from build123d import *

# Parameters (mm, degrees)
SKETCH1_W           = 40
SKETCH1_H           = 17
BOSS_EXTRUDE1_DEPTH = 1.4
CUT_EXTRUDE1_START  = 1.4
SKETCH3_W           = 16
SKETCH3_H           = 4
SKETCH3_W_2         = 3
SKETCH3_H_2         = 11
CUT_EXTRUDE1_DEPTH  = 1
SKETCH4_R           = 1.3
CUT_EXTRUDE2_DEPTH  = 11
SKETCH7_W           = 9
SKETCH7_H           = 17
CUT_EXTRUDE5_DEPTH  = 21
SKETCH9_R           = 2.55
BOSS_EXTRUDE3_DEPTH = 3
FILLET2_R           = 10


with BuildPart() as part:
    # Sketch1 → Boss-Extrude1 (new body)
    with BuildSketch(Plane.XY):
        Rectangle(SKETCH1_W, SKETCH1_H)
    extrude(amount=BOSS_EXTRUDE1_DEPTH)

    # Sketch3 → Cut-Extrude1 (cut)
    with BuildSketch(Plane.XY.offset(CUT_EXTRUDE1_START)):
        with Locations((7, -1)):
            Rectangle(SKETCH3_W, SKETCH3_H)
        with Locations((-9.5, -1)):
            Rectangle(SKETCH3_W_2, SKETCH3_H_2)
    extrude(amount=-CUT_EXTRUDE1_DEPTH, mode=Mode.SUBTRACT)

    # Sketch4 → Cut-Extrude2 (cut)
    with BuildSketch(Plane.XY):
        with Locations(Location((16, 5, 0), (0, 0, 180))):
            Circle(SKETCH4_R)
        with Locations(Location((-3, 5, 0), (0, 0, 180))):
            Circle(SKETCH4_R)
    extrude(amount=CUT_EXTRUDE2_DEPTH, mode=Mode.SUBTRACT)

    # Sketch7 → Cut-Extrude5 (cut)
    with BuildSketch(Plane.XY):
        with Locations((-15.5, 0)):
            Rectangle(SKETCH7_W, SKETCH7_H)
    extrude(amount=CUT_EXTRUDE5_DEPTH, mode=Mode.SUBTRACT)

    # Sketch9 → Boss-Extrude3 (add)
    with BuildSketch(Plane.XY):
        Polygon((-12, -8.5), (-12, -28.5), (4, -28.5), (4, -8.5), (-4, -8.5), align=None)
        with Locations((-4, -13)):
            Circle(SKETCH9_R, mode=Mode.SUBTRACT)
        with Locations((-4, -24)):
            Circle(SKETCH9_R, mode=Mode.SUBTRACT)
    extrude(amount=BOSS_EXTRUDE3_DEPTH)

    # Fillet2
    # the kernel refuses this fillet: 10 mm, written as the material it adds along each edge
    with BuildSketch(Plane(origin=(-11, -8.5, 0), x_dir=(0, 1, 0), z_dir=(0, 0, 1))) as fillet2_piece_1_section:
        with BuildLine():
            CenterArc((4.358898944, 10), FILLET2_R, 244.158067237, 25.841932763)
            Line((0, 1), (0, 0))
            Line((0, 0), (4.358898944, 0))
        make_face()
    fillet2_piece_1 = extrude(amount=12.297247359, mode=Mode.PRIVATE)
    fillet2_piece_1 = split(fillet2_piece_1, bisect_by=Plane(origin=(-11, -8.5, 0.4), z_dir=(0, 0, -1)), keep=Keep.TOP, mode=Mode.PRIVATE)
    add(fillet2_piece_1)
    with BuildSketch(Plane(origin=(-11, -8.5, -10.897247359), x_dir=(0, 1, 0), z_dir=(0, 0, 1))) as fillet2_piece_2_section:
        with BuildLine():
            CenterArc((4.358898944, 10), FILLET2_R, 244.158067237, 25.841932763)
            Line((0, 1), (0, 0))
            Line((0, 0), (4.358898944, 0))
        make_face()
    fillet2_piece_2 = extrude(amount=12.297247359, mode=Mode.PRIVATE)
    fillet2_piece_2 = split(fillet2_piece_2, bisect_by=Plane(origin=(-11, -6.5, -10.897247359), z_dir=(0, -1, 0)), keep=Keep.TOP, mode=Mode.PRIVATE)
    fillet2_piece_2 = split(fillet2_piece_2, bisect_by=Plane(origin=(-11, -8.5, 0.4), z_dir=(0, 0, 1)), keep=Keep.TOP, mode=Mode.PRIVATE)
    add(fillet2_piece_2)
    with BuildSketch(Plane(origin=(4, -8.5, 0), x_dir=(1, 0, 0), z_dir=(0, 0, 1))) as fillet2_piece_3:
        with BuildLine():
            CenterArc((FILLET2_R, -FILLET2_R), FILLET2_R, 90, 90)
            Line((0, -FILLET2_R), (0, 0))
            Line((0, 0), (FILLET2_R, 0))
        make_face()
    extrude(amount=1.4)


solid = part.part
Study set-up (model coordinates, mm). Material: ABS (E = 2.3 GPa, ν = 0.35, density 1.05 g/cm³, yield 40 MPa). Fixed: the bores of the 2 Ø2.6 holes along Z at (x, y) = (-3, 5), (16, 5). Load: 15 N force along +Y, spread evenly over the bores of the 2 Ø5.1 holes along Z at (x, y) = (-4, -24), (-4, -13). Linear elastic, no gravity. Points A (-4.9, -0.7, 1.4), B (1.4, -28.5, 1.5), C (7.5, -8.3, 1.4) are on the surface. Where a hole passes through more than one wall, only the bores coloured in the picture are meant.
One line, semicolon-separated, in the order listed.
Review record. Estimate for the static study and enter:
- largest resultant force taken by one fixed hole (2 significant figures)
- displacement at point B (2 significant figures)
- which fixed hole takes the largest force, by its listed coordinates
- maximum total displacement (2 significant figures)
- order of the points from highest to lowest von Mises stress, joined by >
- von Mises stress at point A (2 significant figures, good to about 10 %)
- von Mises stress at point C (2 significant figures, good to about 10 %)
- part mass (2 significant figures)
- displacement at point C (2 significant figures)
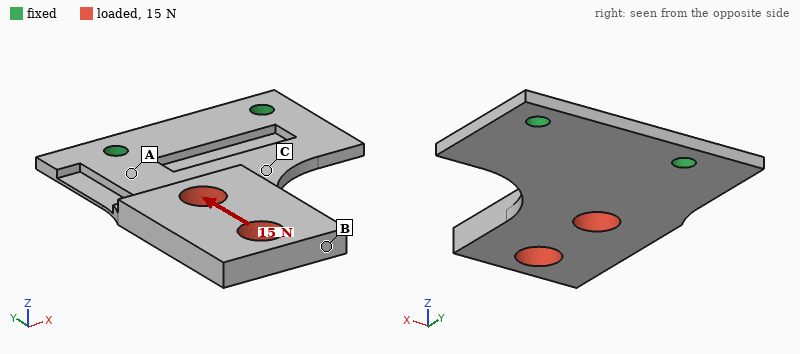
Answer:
15 N; 0.56 mm; (-3, 5); 0.59 mm; A > C > B; 4.3 MPa; 1.6 MPa; 1.6 g; 0.12 mm
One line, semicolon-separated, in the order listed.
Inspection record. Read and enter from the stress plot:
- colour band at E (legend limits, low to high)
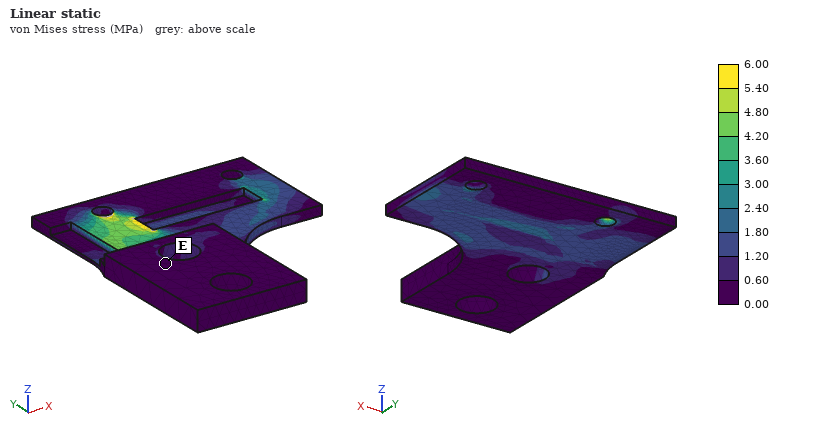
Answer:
0.00 to 0.60 MPa
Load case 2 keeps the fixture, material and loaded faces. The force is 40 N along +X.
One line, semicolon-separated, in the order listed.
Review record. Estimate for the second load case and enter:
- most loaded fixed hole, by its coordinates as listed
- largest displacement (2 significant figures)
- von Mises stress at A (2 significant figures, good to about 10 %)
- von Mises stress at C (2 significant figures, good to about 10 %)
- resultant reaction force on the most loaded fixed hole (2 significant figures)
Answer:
(16, 5); 0.54 mm; 3.5 MPa; 8.7 MPa; 52 N
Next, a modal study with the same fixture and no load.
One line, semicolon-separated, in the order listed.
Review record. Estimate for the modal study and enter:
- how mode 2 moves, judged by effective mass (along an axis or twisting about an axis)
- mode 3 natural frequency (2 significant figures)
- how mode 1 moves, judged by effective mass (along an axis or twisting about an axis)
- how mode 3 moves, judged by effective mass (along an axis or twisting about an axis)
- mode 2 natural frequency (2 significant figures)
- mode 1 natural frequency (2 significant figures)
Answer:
twisting about Y; 2000 Hz; along Z; along Z; 1200 Hz; 230 Hz
